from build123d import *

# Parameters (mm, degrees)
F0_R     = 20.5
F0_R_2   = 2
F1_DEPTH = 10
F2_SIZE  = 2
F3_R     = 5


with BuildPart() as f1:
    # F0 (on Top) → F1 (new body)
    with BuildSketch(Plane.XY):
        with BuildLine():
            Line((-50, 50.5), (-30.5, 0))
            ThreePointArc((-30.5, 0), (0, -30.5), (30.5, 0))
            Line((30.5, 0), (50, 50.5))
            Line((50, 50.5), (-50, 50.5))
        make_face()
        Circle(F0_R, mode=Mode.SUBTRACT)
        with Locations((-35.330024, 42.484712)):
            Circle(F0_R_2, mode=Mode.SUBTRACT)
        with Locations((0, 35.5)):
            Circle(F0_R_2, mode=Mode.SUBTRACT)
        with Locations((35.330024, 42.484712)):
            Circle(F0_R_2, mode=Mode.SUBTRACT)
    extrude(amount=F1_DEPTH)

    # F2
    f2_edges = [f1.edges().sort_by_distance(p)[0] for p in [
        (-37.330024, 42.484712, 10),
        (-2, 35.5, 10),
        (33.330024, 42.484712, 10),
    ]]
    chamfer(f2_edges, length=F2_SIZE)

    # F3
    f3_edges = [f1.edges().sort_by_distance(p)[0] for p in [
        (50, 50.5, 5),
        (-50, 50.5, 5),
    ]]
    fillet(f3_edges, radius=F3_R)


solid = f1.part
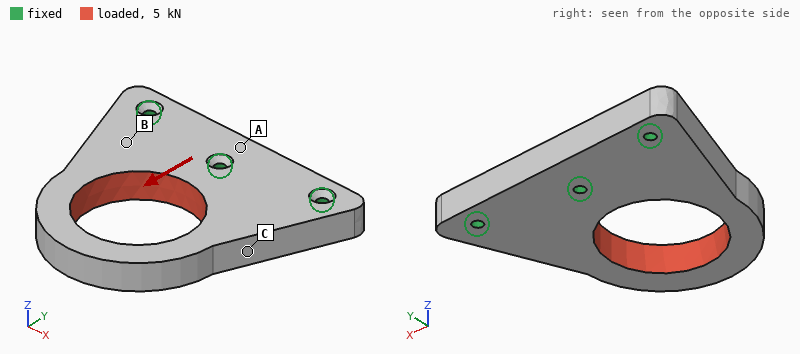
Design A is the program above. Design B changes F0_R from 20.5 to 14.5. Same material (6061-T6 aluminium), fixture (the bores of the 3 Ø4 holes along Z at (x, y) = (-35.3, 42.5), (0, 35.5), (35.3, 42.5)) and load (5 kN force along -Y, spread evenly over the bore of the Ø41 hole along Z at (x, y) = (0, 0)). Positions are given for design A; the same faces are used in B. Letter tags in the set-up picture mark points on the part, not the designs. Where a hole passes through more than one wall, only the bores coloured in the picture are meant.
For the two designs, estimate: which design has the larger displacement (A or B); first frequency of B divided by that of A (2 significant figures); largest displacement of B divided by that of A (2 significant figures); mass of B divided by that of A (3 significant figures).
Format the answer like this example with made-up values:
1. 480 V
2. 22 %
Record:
1. A
2. 0.98
3. 0.60
4. 1.16
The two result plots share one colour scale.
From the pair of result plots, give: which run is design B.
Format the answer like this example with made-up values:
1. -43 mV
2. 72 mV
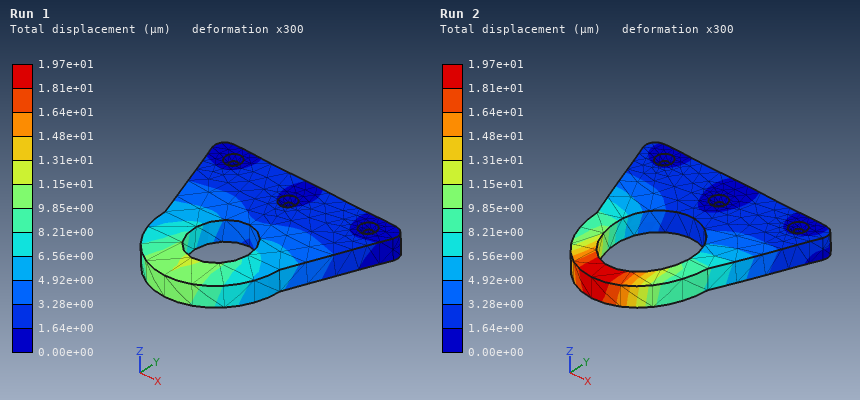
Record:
1. Run 1
